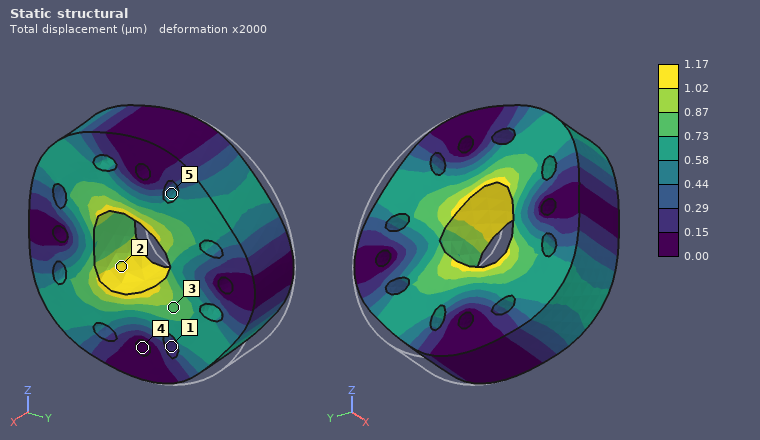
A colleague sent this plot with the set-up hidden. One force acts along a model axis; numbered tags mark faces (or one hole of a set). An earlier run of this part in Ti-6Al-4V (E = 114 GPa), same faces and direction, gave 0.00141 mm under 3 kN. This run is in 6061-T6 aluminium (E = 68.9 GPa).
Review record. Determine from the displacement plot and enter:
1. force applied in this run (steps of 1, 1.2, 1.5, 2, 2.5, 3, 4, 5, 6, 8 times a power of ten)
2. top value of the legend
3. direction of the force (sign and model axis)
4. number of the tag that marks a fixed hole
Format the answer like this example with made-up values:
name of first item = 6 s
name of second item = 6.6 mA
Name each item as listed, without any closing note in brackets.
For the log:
force applied in this run = 1.5 kN
top value of the legend = 1.17 µm
direction of the force = -Y
number of the tag that marks a fixed hole = 4
